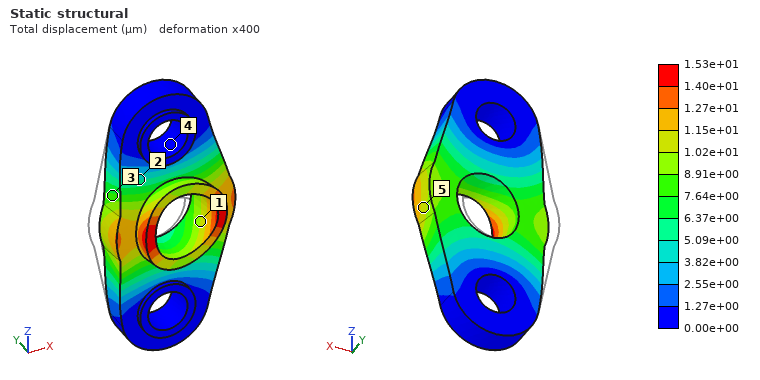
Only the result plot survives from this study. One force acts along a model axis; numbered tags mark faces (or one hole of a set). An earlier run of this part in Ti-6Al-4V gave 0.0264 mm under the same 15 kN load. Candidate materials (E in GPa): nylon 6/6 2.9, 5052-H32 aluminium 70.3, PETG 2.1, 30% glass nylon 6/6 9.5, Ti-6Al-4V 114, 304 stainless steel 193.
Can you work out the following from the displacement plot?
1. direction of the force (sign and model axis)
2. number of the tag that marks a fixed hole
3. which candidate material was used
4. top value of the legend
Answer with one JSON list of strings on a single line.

["+X", "4", "304 stainless steel", "1.53e+01 µm"]
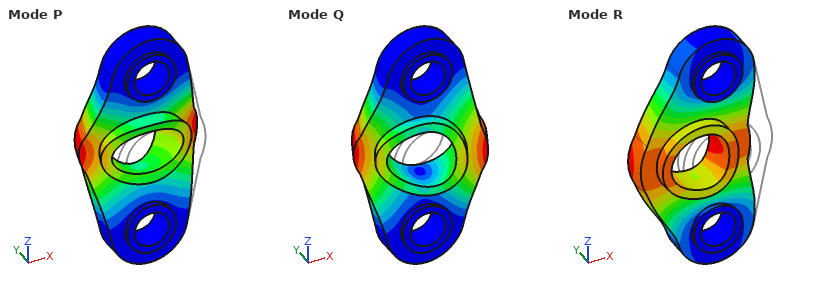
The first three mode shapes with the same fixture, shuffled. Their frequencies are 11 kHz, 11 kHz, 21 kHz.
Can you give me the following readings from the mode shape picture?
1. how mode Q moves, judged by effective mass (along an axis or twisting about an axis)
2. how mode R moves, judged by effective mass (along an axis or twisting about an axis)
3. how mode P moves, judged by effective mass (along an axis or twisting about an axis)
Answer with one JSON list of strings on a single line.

["twisting about Z", "along X", "along Y"]
